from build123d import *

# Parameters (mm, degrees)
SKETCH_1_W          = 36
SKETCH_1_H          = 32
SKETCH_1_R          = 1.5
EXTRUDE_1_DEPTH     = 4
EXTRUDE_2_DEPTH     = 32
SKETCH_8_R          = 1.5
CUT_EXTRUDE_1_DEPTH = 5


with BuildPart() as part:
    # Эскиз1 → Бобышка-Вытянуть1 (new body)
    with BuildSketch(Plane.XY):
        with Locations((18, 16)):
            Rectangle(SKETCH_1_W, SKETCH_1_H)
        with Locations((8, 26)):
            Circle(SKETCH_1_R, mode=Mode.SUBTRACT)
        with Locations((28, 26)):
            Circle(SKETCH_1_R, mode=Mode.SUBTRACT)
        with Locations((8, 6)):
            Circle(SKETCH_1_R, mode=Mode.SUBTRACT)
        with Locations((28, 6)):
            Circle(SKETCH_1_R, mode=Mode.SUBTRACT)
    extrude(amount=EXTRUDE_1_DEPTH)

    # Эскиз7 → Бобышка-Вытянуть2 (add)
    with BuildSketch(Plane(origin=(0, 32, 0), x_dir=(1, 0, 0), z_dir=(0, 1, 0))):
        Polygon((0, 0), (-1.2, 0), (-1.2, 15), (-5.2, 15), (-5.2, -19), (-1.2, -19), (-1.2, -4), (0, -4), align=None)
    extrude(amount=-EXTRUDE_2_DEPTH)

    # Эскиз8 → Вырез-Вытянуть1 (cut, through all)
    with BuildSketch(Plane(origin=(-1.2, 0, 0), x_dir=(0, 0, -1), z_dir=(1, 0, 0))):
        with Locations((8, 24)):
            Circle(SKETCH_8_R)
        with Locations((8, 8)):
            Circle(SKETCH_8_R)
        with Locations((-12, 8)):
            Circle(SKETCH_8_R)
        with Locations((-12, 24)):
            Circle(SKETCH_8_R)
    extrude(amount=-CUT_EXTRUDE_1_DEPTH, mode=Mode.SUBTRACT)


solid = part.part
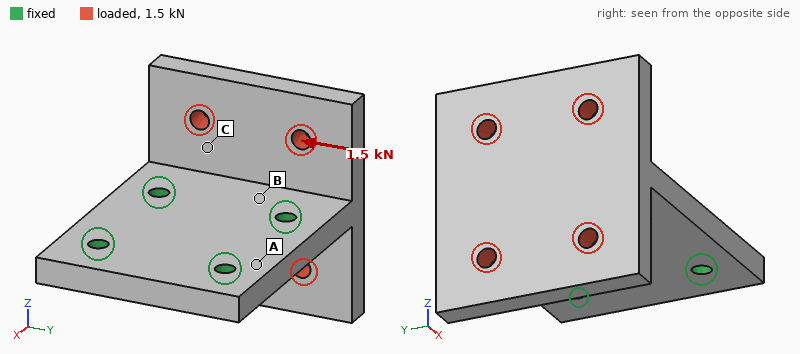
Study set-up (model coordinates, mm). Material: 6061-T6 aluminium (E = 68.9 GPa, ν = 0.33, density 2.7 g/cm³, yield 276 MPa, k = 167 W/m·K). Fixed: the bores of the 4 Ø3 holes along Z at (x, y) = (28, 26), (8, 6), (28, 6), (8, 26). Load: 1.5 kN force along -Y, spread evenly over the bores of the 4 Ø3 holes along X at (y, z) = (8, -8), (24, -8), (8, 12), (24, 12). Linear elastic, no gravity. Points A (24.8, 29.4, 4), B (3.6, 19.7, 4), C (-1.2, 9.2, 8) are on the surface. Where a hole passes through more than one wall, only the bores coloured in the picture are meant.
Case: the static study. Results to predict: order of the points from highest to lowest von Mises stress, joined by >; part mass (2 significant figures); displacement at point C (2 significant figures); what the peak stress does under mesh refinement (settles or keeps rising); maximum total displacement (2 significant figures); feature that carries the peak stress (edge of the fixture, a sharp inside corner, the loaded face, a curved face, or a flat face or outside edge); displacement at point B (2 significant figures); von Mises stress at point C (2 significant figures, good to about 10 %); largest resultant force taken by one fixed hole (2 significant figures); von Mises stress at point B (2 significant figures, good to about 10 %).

B > C > A
24 g
8.0 µm
keeps rising
11 µm
edge of the fixture
2.9 µm
14 MPa
990 N
26 MPa
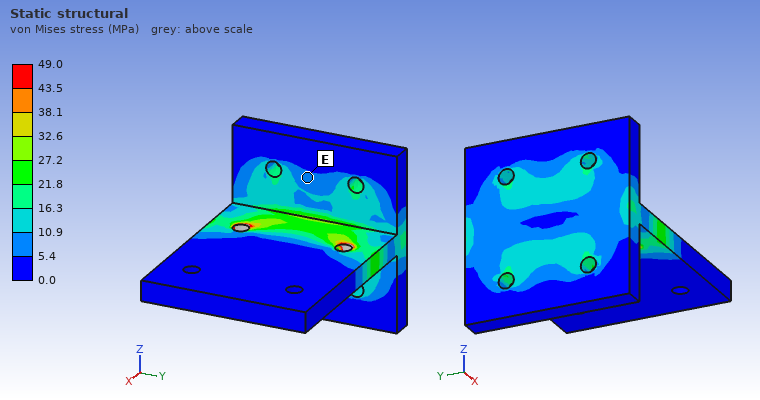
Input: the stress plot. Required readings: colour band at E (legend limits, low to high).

5.4 to 10.9 MPa
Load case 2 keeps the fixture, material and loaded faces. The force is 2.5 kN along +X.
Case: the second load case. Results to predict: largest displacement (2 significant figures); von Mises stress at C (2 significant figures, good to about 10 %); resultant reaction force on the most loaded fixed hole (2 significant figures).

66 µm
56 MPa
1.1 kN
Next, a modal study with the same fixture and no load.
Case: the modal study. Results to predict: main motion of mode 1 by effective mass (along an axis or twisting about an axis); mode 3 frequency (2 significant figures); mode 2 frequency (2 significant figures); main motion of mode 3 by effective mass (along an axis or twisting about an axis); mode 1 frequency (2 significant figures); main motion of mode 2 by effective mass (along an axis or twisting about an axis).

along Z
12 kHz
7900 Hz
along X
4100 Hz
twisting about X
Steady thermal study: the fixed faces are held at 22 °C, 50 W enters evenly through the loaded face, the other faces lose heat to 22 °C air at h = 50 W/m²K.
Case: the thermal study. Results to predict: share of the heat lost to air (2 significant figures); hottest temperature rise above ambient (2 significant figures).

8.9 %
37 K
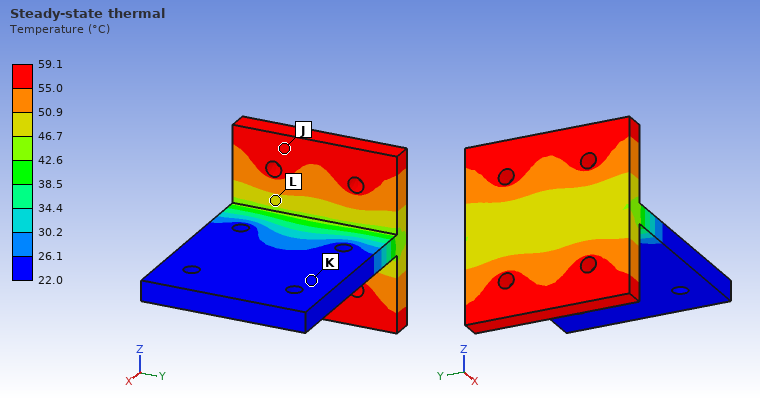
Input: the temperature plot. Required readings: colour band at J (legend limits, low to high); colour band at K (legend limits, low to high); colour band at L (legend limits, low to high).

55.0 to 59.1 °C
22.0 to 26.1 °C
46.7 to 50.9 °C
